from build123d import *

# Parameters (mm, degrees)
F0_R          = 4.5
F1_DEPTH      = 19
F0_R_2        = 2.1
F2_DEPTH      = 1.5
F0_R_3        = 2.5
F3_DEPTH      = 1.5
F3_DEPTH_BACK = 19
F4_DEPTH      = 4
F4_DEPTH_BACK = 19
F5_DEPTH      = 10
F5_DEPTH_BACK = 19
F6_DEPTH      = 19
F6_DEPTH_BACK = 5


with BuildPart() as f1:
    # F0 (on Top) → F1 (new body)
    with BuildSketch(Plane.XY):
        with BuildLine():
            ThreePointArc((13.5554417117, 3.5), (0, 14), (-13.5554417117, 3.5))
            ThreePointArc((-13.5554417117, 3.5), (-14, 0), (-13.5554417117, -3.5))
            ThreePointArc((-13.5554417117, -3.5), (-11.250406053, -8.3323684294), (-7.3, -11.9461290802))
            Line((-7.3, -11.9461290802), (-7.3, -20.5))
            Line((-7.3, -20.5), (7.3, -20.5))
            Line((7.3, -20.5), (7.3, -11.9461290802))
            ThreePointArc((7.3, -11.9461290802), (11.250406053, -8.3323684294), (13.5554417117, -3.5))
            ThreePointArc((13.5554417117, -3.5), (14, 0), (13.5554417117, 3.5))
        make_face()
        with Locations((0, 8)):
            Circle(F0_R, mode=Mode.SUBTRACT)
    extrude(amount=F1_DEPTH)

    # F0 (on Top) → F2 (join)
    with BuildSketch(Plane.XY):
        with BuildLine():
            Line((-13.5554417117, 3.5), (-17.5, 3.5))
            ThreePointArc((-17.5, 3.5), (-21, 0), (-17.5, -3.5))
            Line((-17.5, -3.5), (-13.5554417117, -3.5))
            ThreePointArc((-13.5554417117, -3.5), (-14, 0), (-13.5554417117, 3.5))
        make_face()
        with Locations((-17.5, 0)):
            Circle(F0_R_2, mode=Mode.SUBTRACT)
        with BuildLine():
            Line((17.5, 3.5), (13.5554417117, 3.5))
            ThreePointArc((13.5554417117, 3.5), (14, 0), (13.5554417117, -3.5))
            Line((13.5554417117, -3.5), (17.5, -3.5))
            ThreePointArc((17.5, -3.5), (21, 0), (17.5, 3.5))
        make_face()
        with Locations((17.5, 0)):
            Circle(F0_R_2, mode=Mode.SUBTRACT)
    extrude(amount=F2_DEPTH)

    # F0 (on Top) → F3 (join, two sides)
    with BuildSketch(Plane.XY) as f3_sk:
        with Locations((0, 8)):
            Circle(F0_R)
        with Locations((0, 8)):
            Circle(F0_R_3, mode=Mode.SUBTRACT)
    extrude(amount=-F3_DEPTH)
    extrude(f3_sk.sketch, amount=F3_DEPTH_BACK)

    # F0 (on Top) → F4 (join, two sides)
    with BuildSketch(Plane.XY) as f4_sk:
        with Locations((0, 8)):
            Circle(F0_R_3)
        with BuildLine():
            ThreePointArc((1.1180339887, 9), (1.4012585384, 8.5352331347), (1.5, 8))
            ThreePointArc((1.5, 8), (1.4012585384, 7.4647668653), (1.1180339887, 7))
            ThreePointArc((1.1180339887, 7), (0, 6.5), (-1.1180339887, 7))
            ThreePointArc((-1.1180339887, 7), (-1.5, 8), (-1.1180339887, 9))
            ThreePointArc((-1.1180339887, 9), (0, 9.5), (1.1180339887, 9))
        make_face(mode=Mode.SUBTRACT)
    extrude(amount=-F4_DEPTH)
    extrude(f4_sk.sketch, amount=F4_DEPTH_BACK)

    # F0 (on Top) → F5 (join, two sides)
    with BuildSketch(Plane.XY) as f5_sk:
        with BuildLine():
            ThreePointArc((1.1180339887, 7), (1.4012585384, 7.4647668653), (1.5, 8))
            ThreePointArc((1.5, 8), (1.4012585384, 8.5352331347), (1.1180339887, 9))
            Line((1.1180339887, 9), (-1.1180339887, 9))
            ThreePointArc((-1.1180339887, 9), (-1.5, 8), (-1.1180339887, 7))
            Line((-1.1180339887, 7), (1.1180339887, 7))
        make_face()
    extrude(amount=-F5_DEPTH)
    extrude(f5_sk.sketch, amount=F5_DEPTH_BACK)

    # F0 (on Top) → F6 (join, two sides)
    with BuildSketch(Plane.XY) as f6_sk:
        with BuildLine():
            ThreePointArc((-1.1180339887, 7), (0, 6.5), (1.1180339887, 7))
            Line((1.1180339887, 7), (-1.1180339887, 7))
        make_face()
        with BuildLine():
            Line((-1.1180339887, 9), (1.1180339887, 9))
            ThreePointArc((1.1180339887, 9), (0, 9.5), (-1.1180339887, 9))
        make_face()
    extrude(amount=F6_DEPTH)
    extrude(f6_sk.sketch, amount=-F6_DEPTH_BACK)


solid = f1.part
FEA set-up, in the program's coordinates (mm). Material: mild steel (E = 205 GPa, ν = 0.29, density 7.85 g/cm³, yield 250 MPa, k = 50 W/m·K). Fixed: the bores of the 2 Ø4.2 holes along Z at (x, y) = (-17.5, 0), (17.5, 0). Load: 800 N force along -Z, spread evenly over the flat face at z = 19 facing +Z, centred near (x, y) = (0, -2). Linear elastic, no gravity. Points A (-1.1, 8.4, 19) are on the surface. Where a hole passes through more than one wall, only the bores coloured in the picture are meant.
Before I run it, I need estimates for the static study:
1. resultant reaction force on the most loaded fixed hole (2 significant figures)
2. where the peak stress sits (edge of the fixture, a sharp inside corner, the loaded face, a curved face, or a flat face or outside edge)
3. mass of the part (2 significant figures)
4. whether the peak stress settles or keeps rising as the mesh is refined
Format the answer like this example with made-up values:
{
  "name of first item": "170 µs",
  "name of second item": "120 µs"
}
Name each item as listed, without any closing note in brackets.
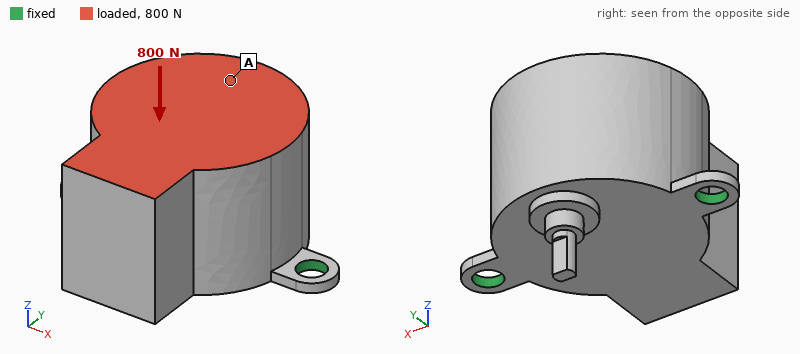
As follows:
{
  "resultant reaction force on the most loaded fixed hole": "460 N",
  "where the peak stress sits": "edge of the fixture",
  "mass of the part": "110 g",
  "whether the peak stress settles or keeps rising as the mesh is refined": "keeps rising"
}
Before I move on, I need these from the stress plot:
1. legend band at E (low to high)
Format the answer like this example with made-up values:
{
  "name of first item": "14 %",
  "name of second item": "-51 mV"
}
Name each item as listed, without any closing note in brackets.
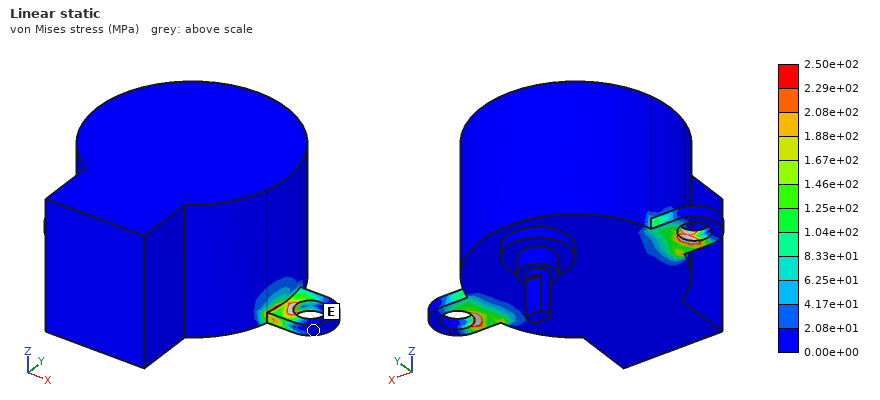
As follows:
{
  "legend band at E": "0.00e+00 to 2.08e+01 MPa"
}
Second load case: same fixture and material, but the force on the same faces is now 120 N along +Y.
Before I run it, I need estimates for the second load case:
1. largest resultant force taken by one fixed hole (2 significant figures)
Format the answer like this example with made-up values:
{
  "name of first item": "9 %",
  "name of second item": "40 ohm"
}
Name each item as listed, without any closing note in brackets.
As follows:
{
  "largest resultant force taken by one fixed hole": "60 N"
}
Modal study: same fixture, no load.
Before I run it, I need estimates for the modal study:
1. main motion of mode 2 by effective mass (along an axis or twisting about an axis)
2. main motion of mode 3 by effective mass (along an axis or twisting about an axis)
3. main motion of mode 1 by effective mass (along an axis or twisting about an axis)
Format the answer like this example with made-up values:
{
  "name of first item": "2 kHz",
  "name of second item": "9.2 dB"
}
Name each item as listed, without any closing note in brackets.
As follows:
{
  "main motion of mode 2 by effective mass": "along Z",
  "main motion of mode 3 by effective mass": "along X",
  "main motion of mode 1 by effective mass": "along Y"
}
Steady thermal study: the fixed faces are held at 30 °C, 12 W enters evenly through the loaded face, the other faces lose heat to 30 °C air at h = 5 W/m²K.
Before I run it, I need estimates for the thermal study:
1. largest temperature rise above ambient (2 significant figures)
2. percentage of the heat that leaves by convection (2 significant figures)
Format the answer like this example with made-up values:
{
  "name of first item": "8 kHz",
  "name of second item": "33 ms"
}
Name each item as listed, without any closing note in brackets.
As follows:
{
  "largest temperature rise above ambient": "49 K",
  "percentage of the heat that leaves by convection": "5.2 %"
}
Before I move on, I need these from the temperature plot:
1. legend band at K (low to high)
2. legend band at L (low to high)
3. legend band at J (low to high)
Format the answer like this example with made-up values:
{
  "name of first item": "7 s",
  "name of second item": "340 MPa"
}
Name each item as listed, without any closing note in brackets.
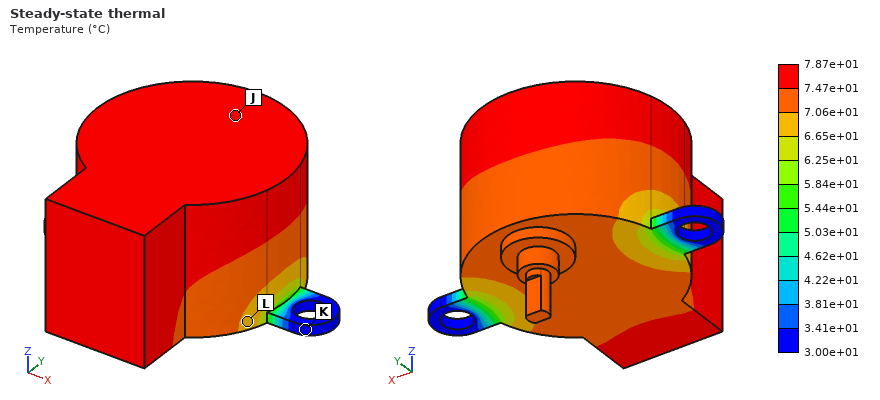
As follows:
{
  "legend band at K": "3.00e+01 to 3.41e+01 °C",
  "legend band at L": "6.65e+01 to 7.06e+01 °C",
  "legend band at J": "7.47e+01 to 7.87e+01 °C"
}
